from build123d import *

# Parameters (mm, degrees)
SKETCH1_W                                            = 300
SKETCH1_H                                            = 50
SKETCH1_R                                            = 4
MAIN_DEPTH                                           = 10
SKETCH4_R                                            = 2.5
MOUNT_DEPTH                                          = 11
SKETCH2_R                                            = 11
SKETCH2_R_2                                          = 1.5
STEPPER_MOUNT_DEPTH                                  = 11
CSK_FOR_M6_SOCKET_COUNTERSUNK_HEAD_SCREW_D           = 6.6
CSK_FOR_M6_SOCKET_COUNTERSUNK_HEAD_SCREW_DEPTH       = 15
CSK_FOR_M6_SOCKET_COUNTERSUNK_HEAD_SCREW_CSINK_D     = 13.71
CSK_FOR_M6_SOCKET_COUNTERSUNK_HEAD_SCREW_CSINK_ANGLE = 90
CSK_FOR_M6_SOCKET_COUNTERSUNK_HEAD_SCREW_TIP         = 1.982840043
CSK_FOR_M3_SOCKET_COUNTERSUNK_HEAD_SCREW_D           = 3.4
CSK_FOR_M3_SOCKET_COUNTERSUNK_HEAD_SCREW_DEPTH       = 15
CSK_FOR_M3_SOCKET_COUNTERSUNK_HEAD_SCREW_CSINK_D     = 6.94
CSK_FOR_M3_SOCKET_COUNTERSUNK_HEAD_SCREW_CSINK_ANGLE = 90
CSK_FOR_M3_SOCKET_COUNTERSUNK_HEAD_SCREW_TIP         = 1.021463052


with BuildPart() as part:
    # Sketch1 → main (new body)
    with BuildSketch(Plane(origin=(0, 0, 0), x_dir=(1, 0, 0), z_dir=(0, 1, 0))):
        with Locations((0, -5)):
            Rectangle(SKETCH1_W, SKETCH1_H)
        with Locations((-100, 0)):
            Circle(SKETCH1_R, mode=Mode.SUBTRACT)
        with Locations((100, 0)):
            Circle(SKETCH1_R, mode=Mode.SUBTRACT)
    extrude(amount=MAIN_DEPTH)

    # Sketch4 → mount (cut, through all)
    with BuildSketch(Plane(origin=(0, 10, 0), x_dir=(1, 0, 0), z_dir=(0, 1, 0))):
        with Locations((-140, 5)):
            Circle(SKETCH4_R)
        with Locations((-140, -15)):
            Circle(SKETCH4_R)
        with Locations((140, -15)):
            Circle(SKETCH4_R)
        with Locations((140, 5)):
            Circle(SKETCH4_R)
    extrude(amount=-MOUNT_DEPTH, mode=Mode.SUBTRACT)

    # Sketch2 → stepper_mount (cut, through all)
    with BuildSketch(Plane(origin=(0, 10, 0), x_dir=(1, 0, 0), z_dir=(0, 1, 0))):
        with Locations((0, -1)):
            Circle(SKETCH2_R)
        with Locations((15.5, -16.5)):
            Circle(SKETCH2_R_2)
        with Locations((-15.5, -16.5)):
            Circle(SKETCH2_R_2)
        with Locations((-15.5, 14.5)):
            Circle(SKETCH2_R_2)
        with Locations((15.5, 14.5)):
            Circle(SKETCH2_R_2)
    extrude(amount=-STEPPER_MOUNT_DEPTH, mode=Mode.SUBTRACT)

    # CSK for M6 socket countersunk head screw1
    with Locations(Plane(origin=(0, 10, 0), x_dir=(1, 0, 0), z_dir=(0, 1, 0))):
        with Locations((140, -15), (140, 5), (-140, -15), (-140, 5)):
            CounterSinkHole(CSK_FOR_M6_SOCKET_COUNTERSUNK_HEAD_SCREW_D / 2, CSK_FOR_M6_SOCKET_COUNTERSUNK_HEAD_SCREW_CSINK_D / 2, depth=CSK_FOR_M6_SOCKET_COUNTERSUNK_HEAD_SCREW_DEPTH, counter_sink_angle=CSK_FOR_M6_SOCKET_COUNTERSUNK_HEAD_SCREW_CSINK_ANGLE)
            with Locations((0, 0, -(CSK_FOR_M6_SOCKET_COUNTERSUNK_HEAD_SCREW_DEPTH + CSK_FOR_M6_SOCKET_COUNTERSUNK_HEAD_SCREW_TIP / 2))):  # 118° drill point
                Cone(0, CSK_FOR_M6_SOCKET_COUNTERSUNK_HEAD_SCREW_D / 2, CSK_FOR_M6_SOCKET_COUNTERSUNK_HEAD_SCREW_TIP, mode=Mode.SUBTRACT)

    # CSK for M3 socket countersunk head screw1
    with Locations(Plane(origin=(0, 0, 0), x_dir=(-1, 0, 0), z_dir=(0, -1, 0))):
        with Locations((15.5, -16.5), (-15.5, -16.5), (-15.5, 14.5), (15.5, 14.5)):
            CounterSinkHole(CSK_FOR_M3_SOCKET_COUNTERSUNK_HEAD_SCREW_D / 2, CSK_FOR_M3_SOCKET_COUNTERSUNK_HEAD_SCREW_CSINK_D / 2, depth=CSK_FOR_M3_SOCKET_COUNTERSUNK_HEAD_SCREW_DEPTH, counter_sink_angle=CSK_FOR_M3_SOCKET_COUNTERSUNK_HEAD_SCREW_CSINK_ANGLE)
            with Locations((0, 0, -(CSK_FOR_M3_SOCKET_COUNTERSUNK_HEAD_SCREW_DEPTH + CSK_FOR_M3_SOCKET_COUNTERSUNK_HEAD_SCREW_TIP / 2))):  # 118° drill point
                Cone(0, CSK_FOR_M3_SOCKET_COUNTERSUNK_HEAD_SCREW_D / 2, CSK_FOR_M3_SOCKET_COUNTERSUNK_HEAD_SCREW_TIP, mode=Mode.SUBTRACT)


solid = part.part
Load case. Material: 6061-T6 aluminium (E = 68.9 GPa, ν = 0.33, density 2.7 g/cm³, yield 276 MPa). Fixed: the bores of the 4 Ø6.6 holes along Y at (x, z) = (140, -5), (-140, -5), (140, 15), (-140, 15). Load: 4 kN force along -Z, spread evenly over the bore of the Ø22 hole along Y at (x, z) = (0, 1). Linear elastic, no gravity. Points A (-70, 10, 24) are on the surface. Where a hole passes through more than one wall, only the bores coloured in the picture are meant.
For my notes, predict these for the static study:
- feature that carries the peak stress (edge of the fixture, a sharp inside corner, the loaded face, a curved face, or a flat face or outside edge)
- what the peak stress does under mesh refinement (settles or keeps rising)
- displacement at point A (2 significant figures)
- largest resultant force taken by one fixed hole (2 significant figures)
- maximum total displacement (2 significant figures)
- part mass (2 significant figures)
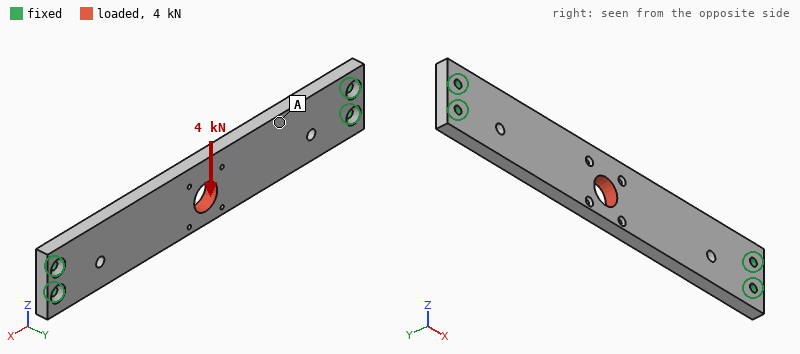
edge of the fixture
keeps rising
0.067 mm
5.1 kN
0.12 mm
390 g
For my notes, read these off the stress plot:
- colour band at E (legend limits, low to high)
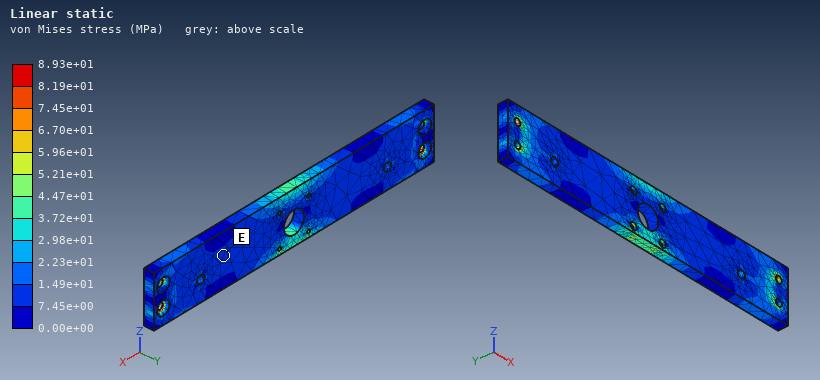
7.45e+00 to 1.49e+01 MPa
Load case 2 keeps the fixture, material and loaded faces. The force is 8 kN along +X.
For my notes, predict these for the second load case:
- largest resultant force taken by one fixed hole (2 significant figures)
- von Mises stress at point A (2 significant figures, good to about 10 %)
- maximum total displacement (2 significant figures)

2.2 kN
6.4 MPa
20 µm
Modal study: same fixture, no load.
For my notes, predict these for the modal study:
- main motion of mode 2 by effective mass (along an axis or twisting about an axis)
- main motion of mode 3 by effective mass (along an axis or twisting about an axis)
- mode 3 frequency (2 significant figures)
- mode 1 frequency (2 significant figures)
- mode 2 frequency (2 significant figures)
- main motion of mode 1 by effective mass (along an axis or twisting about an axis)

twisting about Z
twisting about X
2100 Hz
610 Hz
1700 Hz
along Y
